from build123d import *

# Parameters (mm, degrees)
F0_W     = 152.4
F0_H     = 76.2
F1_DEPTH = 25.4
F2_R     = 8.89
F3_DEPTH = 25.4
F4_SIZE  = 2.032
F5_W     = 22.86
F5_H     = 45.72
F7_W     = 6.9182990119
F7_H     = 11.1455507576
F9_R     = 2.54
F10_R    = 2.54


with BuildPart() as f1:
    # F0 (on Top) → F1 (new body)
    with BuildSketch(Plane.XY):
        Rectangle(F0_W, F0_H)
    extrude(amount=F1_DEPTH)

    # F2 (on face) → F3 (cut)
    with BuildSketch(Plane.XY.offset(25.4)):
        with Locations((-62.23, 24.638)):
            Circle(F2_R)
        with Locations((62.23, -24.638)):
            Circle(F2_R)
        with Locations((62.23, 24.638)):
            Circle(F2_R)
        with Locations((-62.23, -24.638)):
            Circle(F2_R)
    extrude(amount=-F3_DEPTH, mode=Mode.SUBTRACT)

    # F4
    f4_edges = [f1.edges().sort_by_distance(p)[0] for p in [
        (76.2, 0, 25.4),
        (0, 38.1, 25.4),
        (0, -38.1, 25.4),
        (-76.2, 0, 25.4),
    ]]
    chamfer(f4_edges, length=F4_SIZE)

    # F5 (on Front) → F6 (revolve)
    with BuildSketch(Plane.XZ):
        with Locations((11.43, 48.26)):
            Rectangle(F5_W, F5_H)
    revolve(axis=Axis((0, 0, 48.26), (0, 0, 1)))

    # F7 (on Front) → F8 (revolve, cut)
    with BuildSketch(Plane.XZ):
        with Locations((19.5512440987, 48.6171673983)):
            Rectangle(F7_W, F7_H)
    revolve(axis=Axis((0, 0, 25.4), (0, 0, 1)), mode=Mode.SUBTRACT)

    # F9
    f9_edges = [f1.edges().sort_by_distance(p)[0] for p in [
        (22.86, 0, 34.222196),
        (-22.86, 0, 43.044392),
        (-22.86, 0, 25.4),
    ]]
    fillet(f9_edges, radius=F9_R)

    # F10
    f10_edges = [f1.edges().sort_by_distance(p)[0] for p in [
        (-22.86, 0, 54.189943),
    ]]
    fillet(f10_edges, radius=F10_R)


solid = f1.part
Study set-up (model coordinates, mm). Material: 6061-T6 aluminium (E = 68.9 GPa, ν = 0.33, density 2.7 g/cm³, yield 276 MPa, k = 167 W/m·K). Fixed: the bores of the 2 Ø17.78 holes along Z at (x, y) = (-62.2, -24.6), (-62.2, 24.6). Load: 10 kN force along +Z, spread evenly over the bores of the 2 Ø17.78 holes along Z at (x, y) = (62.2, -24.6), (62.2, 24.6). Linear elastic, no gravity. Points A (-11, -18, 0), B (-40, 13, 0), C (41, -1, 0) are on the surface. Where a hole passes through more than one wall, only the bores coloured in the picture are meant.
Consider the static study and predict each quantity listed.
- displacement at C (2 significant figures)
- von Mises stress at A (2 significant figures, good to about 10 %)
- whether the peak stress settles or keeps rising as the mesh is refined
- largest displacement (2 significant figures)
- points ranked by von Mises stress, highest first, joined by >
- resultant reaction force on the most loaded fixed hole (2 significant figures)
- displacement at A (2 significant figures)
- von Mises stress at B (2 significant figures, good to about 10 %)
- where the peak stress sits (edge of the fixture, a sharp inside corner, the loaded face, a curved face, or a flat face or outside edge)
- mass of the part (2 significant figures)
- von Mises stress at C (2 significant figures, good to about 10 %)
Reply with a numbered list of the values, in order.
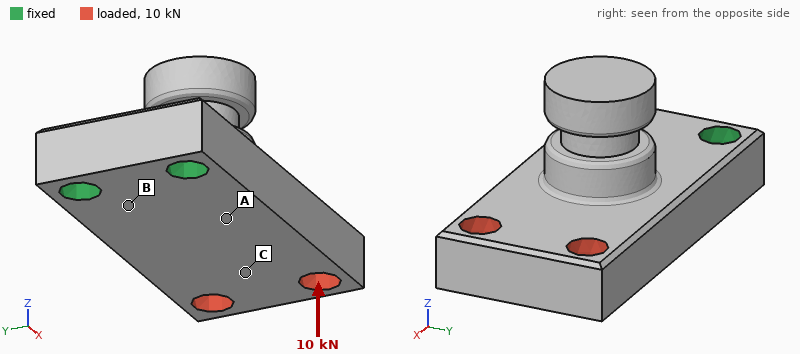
1. 0.57 mm
2. 72 MPa
3. keeps rising
4. 0.89 mm
5. B > A > C
6. 5.1 kN
7. 0.19 mm
8. 110 MPa
9. edge of the fixture
10. 900 g
11. 26 MPa
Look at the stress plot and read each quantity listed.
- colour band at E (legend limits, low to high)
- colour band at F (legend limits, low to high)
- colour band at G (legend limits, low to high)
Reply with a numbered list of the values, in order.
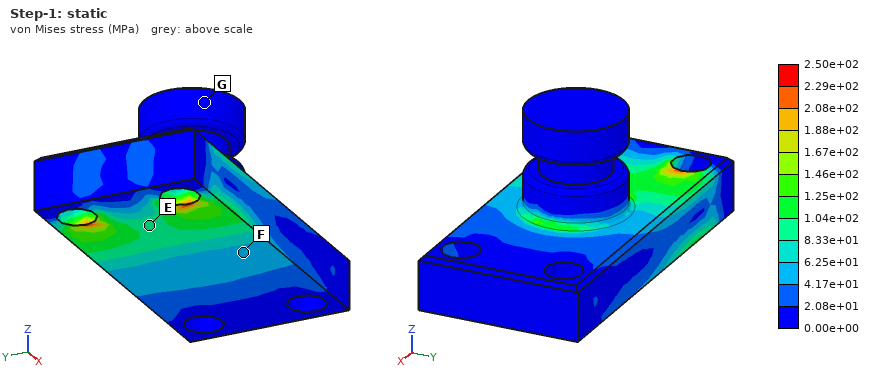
1. 8.33e+01 to 1.04e+02 MPa
2. 4.17e+01 to 6.25e+01 MPa
3. 0.00e+00 to 2.08e+01 MPa
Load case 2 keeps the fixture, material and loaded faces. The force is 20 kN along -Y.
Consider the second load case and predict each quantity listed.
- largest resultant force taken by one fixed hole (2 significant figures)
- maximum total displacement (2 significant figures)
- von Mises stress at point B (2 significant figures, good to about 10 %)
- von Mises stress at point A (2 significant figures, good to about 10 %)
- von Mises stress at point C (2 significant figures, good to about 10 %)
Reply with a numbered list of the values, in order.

1. 44 kN
2. 0.28 mm
3. 38 MPa
4. 37 MPa
5. 23 MPa
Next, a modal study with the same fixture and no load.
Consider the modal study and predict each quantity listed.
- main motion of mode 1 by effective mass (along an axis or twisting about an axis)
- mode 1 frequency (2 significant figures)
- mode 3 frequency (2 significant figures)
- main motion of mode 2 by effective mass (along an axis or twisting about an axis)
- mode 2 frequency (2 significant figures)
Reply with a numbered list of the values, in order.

1. along Z
2. 1100 Hz
3. 3400 Hz
4. along Y
5. 2800 Hz
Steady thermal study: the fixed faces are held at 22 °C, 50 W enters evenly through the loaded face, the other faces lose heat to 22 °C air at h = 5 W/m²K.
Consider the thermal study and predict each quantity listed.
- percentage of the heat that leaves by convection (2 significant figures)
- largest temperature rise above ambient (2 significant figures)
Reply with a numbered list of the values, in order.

1. 3.4 %
2. 20 K
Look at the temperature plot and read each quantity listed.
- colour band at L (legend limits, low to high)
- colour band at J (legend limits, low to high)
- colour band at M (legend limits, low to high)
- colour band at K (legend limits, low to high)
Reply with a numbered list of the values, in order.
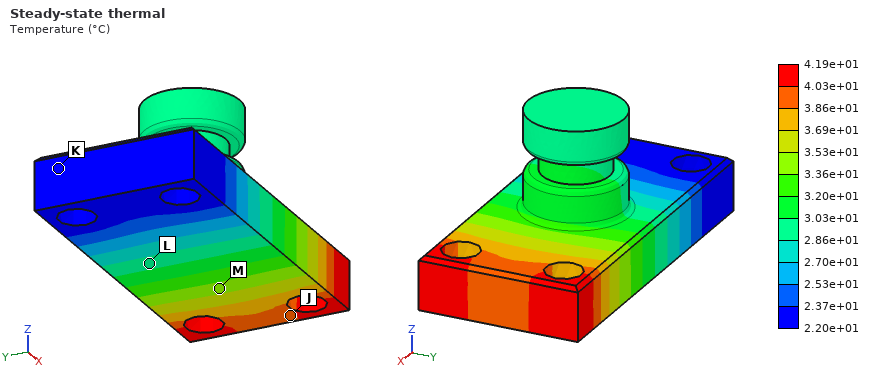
1. 2.86e+01 to 3.03e+01 °C
2. 3.86e+01 to 4.03e+01 °C
3. 3.36e+01 to 3.53e+01 °C
4. 2.20e+01 to 2.37e+01 °C
